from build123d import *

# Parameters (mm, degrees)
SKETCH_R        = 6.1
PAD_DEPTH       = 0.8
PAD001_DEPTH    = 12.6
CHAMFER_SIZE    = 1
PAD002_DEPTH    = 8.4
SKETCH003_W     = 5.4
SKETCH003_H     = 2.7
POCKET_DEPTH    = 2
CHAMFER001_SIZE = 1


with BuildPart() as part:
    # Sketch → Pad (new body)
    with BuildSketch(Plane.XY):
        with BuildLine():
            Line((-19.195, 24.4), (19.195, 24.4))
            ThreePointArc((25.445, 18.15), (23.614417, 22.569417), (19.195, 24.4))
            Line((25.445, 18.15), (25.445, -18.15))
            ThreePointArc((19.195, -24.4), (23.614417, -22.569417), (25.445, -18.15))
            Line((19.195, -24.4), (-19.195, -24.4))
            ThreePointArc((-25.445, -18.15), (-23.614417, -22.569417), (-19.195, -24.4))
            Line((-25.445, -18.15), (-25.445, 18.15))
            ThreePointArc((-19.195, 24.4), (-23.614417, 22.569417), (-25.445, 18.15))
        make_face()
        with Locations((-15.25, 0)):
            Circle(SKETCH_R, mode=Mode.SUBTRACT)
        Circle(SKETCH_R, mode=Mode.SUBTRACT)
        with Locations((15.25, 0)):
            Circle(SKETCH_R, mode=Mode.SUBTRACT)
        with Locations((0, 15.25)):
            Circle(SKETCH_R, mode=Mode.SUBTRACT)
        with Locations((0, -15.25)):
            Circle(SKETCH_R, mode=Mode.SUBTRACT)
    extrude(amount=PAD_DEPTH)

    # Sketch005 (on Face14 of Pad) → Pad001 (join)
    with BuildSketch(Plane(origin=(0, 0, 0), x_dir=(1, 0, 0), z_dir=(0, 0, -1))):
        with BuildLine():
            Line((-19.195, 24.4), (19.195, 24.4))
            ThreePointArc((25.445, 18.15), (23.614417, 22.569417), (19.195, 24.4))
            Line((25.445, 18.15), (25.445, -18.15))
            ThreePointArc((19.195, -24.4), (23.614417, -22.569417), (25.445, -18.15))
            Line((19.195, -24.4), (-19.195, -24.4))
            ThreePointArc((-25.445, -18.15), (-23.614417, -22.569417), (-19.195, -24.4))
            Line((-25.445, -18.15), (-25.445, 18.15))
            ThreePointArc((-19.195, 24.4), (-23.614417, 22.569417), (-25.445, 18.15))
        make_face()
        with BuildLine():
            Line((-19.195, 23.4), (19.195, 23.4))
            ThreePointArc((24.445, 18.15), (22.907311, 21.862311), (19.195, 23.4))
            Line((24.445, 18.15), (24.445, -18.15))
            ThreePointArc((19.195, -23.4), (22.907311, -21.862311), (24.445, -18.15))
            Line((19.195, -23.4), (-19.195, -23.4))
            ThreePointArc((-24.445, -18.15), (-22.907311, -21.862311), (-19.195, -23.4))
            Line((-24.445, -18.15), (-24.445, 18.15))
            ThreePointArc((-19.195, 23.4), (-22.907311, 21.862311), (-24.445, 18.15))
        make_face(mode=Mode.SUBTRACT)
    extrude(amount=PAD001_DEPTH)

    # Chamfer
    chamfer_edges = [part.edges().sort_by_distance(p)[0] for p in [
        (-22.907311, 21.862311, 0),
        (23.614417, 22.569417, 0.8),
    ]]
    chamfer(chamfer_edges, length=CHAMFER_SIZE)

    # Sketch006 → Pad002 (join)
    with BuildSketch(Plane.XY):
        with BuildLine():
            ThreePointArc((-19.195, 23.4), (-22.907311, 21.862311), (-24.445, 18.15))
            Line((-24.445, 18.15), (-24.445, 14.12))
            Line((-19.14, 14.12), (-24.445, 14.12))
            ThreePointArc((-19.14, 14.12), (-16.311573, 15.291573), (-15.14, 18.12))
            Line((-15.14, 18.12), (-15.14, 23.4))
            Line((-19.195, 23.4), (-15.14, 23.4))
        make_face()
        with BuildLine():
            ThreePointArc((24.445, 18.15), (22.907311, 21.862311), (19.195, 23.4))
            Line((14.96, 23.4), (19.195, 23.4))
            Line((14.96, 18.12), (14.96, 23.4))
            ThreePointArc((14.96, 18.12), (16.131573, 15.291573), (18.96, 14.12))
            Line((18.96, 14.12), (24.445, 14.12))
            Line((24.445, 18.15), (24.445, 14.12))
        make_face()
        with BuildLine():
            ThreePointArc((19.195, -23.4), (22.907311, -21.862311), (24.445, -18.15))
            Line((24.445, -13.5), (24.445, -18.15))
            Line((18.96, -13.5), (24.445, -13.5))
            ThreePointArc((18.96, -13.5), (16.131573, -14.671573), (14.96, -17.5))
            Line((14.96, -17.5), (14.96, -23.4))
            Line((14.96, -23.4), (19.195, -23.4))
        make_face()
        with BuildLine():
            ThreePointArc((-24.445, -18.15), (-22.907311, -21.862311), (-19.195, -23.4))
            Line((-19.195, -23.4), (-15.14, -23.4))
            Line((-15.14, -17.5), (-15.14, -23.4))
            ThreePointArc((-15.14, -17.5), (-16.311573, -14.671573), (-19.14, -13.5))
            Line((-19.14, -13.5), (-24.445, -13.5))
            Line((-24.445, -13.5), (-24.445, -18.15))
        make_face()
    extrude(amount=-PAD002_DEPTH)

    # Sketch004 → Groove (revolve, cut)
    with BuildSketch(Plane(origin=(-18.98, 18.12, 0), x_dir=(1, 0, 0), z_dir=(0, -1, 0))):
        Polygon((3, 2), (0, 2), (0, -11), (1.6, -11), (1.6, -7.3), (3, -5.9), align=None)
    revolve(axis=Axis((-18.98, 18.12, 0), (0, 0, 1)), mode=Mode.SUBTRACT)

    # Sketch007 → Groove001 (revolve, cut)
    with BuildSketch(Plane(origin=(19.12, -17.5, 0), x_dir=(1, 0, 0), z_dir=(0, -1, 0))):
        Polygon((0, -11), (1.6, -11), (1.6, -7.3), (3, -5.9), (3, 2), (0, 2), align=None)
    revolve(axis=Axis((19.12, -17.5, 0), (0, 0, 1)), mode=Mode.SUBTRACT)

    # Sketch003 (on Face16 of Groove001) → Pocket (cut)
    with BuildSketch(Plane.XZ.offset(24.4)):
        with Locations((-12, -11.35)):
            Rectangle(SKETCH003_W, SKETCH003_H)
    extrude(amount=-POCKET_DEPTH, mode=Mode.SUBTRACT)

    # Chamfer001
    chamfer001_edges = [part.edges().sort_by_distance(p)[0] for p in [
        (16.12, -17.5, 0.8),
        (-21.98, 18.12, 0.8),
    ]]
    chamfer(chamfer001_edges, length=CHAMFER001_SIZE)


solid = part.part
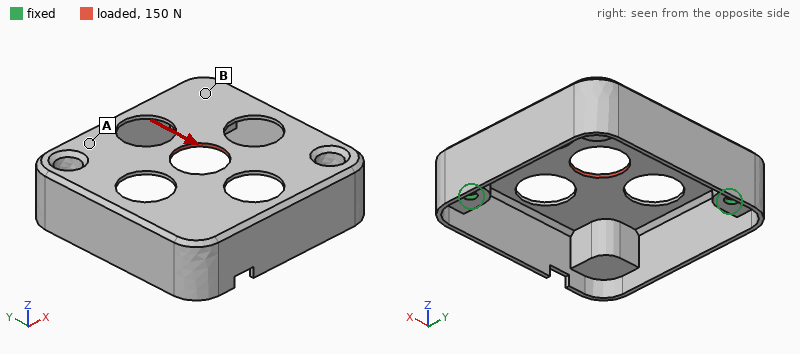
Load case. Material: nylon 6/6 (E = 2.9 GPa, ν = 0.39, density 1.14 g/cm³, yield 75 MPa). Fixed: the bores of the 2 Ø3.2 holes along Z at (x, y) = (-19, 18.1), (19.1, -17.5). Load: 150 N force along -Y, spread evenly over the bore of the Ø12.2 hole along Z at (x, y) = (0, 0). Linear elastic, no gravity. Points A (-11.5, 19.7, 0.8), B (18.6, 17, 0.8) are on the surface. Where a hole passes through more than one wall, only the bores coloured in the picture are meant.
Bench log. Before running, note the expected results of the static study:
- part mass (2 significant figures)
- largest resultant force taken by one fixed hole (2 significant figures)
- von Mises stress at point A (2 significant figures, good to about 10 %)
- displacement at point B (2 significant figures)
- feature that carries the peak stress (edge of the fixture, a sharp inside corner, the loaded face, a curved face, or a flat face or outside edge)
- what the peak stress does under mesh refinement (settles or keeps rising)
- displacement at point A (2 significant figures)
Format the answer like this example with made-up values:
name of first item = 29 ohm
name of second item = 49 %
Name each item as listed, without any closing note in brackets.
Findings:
part mass = 6.9 g
largest resultant force taken by one fixed hole = 76 N
von Mises stress at point A = 8.0 MPa
displacement at point B = 0.64 mm
feature that carries the peak stress = edge of the fixture
what the peak stress does under mesh refinement = keeps rising
displacement at point A = 0.27 mm
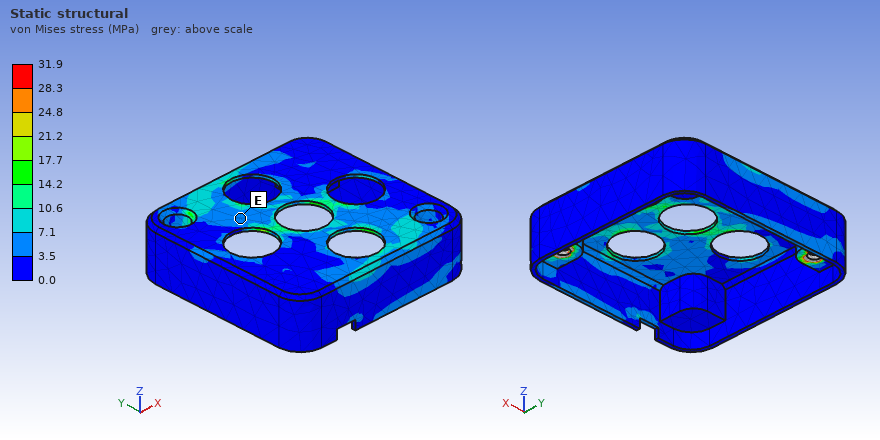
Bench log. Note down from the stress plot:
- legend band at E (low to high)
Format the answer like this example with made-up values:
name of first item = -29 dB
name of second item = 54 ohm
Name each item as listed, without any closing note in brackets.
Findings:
legend band at E = 3.5 to 7.1 MPa
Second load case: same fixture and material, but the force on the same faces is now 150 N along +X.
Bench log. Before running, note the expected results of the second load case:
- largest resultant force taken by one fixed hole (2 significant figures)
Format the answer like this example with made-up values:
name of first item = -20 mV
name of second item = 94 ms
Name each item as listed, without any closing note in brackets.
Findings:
largest resultant force taken by one fixed hole = 76 N
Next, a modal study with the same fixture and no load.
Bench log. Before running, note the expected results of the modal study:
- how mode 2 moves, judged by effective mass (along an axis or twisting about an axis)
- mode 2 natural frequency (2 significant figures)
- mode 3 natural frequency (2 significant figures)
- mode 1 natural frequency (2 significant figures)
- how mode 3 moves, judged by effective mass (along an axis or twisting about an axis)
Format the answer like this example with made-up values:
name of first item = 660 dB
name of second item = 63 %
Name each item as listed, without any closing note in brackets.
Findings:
how mode 2 moves, judged by effective mass = along Z
mode 2 natural frequency = 1000 Hz
mode 3 natural frequency = 1200 Hz
mode 1 natural frequency = 580 Hz
how mode 3 moves, judged by effective mass = along Z
